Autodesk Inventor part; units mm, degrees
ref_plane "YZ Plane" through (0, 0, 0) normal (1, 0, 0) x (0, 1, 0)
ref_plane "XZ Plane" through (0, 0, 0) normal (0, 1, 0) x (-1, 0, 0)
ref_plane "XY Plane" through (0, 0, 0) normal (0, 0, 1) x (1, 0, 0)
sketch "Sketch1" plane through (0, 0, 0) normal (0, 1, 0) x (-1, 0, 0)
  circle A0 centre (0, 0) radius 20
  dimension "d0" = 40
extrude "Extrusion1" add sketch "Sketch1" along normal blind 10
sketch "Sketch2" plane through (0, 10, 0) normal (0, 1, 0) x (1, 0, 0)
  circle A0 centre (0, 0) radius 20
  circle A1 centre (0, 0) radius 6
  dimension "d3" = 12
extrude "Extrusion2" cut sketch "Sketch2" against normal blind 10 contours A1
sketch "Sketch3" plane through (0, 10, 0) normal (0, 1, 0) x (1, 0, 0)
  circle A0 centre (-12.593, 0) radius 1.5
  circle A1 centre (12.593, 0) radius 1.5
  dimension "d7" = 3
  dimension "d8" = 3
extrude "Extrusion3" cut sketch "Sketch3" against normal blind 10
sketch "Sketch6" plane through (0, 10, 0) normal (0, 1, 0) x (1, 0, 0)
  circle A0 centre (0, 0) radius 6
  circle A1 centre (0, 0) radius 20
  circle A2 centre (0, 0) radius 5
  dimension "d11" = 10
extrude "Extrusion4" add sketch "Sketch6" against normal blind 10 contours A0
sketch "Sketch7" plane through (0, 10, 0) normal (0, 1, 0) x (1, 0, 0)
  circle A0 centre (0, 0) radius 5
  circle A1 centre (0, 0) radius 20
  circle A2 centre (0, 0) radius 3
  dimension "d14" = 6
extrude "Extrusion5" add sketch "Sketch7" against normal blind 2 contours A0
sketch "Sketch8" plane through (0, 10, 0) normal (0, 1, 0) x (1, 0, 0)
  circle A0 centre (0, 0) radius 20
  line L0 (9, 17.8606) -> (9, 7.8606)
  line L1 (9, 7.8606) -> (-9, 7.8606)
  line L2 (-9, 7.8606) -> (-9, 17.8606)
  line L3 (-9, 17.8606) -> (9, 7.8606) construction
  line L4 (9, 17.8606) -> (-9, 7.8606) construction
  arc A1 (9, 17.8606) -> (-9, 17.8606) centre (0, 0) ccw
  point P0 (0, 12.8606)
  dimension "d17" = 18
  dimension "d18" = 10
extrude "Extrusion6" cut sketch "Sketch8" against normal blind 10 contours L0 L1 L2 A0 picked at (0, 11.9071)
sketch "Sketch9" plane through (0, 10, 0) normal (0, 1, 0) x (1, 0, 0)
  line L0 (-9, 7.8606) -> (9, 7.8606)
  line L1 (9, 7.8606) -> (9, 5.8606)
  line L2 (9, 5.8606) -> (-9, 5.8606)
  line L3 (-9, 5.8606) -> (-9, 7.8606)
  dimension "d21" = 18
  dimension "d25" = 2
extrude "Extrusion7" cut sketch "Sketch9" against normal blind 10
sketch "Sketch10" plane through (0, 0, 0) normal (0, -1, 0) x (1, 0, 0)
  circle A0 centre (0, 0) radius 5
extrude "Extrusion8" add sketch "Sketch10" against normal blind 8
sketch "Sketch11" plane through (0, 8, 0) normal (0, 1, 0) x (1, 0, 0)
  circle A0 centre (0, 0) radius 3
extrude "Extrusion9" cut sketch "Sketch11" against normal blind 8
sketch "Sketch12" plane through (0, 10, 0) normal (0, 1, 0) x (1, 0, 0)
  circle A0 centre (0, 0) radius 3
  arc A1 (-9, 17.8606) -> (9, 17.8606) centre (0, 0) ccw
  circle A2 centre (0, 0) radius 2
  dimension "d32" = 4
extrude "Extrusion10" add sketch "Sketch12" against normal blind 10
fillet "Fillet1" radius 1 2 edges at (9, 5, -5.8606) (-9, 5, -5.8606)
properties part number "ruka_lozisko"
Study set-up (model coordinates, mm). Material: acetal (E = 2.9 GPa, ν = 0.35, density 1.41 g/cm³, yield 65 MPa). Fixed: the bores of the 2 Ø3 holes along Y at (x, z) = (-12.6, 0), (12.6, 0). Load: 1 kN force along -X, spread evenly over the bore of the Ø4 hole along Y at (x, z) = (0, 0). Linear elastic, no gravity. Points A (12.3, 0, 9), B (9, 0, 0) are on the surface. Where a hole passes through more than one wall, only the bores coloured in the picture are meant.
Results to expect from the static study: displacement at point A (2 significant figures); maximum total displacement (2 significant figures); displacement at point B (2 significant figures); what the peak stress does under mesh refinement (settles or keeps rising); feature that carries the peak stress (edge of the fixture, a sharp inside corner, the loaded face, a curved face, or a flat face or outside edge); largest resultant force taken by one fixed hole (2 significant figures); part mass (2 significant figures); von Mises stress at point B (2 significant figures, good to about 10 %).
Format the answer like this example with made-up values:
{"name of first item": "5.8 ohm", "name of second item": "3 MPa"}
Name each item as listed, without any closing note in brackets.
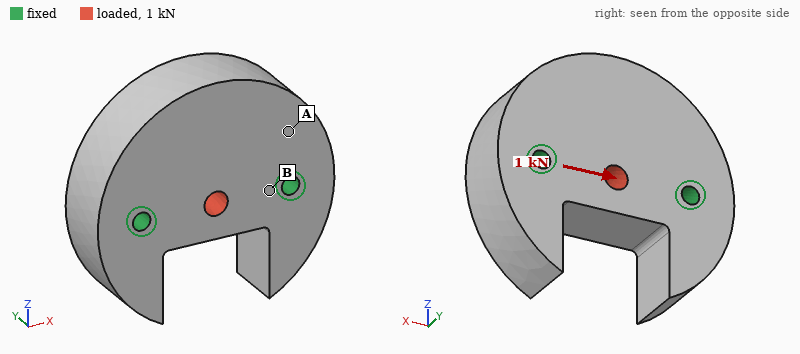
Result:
{"displacement at point A": "8.9 µm", "maximum total displacement": "24 µm", "displacement at point B": "6.3 µm", "what the peak stress does under mesh refinement": "keeps rising", "feature that carries the peak stress": "edge of the fixture", "largest resultant force taken by one fixed hole": "500 N", "part mass": "14 g", "von Mises stress at point B": "7.0 MPa"}
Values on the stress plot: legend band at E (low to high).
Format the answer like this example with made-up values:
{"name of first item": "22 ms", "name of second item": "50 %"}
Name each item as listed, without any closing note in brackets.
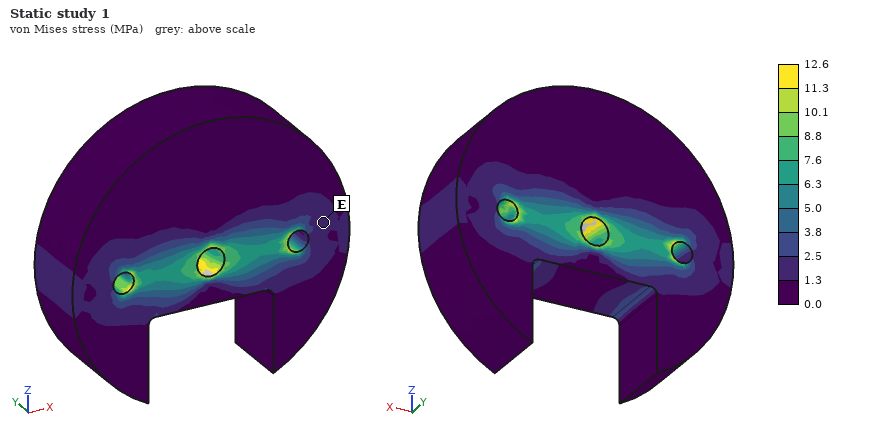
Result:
{"legend band at E": "1.3 to 2.5 MPa"}
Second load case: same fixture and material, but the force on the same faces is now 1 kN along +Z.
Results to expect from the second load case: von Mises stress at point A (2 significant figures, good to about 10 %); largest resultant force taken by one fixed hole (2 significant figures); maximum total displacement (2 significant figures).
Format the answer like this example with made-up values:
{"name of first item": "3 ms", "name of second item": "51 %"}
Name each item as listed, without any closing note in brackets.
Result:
{"von Mises stress at point A": "3.0 MPa", "largest resultant force taken by one fixed hole": "510 N", "maximum total displacement": "56 µm"}
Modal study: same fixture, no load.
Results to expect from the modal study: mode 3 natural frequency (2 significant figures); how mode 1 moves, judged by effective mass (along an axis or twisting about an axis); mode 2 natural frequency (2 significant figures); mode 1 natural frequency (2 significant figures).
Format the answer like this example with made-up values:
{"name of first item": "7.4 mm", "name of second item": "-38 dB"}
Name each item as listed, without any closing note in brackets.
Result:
{"mode 3 natural frequency": "8600 Hz", "how mode 1 moves, judged by effective mass": "along Y", "mode 2 natural frequency": "8600 Hz", "mode 1 natural frequency": "4700 Hz"}
